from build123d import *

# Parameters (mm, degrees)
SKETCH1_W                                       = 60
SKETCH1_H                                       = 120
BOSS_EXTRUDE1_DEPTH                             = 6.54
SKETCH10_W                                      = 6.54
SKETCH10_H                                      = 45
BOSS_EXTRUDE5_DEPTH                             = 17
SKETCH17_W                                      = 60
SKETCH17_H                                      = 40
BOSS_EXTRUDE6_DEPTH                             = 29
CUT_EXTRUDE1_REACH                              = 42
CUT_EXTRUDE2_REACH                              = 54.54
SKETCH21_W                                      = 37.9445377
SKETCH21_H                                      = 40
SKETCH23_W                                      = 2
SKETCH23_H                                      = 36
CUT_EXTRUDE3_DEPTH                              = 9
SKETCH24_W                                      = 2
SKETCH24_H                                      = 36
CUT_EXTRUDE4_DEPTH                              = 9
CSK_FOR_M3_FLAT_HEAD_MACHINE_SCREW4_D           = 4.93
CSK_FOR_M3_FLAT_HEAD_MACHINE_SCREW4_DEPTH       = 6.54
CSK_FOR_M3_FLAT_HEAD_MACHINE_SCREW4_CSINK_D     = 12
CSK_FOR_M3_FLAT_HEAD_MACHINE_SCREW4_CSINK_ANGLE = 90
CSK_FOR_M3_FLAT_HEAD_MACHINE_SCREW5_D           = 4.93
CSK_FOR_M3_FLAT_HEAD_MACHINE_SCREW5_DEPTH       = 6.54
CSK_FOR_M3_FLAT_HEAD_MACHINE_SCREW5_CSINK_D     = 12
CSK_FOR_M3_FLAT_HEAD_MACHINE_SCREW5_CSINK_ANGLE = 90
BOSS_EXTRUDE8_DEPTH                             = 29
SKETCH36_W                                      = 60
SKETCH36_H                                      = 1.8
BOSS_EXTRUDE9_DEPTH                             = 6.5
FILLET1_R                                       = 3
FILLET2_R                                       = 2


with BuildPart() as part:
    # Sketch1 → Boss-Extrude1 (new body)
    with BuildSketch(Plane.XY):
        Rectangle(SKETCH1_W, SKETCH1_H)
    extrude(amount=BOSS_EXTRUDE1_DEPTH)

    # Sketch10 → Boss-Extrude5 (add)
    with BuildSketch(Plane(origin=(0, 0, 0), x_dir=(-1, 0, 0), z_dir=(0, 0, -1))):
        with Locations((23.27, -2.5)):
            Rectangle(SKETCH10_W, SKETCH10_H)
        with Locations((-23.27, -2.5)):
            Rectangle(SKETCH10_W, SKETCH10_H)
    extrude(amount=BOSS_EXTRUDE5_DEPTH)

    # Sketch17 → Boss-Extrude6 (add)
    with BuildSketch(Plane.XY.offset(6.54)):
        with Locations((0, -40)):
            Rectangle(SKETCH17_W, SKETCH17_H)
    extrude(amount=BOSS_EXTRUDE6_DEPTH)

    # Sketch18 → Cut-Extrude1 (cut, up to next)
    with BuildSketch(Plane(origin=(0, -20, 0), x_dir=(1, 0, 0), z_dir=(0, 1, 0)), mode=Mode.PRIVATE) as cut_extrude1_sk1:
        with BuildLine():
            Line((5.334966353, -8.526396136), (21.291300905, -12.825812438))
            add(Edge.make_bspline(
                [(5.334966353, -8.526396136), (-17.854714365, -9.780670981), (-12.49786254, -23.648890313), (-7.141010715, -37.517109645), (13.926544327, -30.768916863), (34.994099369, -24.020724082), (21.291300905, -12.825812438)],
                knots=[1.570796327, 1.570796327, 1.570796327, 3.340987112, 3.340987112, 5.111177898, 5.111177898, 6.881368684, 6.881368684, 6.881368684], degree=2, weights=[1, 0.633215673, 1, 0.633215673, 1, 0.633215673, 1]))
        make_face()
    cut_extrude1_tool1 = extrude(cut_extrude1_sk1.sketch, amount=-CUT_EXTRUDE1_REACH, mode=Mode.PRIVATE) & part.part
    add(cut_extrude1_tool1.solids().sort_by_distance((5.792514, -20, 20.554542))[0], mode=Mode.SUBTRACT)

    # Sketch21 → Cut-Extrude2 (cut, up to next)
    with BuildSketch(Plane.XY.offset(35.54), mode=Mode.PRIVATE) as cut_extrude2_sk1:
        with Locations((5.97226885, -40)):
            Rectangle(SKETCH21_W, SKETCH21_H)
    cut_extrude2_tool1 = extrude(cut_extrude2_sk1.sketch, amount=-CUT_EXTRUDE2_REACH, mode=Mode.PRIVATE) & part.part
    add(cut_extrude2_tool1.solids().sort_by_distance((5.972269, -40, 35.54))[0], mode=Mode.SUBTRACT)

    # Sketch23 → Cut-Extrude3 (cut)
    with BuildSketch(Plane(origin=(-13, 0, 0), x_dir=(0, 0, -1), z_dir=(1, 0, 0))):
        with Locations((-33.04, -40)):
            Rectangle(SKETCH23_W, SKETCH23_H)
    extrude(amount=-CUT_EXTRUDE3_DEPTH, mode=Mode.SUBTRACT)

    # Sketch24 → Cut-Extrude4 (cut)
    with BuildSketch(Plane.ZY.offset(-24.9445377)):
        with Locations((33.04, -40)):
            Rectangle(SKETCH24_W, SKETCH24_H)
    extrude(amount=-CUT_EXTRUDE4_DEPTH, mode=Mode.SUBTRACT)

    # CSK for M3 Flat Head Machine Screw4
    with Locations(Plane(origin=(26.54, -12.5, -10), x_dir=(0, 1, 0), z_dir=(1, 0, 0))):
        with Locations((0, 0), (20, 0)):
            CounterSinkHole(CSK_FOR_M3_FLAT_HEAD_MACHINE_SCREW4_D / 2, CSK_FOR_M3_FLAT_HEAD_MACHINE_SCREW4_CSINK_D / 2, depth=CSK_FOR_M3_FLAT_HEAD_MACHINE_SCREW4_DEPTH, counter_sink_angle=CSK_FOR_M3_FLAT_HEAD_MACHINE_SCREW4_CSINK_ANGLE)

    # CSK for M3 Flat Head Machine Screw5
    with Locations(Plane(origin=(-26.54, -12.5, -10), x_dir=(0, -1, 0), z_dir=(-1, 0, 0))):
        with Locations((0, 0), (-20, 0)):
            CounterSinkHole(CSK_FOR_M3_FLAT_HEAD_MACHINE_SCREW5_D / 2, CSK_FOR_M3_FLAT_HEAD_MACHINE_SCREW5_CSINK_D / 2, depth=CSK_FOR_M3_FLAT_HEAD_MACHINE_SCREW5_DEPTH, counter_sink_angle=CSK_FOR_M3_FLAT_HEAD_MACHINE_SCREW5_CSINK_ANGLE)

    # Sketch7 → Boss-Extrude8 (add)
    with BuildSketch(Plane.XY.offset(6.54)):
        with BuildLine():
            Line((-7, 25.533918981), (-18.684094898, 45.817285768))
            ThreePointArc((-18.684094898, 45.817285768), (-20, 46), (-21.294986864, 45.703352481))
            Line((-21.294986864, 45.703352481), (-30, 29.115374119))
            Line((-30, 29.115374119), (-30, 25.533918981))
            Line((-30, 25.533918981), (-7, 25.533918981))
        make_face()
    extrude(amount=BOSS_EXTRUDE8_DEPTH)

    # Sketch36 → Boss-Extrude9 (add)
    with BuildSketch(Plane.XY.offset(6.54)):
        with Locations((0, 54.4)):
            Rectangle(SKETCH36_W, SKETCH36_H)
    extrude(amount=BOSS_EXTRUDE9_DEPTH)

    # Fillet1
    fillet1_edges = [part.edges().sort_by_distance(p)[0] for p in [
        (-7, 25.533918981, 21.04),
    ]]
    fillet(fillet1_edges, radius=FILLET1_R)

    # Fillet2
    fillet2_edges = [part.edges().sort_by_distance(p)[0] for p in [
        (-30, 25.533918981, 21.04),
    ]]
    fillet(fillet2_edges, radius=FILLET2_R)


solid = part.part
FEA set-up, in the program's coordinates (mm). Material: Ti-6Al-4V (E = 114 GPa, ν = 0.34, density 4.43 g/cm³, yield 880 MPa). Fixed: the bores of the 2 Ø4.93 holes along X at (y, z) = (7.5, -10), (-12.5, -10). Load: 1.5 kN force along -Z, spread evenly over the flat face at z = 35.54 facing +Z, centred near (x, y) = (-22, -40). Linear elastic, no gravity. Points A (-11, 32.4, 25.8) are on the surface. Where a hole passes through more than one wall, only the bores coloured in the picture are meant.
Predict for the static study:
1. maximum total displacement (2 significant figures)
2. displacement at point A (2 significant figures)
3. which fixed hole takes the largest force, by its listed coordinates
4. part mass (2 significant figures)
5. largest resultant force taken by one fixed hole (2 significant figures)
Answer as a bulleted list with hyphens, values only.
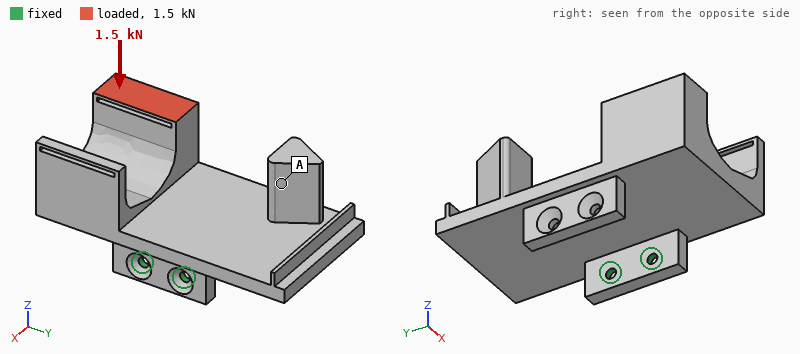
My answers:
- 1.2 mm
- 0.53 mm
- (-12.5, -10)
- 430 g
- 3.2 kN
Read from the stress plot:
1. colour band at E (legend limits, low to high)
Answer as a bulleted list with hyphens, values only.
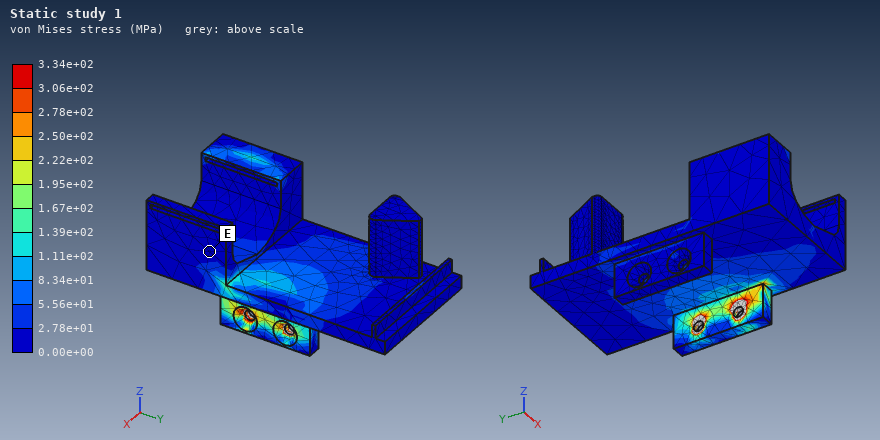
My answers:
- 0.00e+00 to 2.78e+01 MPa
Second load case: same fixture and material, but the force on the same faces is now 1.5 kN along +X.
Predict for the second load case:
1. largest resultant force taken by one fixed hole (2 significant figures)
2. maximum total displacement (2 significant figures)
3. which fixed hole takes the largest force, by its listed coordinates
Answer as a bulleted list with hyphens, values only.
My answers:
- 3.1 kN
- 1.2 mm
- (-12.5, -10)
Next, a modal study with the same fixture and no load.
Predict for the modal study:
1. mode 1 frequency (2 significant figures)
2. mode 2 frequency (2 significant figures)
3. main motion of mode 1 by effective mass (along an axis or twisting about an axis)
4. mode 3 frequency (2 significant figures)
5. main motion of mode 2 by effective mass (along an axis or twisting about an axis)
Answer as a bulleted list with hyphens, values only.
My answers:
- 440 Hz
- 830 Hz
- along Z
- 980 Hz
- along Y
